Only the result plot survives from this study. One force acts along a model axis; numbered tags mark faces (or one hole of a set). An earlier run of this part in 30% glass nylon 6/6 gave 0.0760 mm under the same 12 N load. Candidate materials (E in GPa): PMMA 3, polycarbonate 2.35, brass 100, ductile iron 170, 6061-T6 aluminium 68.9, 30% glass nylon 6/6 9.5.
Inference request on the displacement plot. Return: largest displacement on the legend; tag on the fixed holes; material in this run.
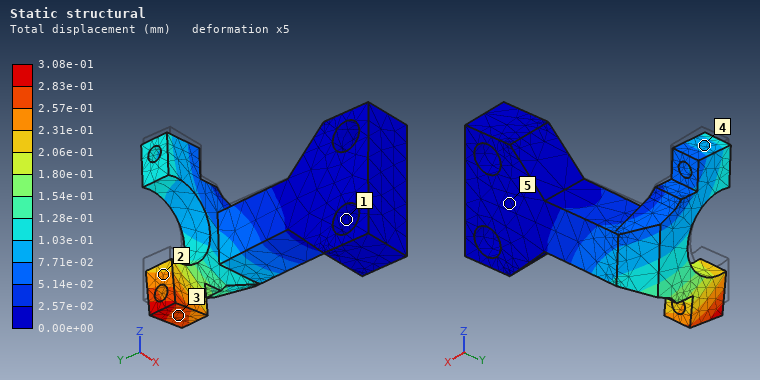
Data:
3.08e-01 mm
1
polycarbonate
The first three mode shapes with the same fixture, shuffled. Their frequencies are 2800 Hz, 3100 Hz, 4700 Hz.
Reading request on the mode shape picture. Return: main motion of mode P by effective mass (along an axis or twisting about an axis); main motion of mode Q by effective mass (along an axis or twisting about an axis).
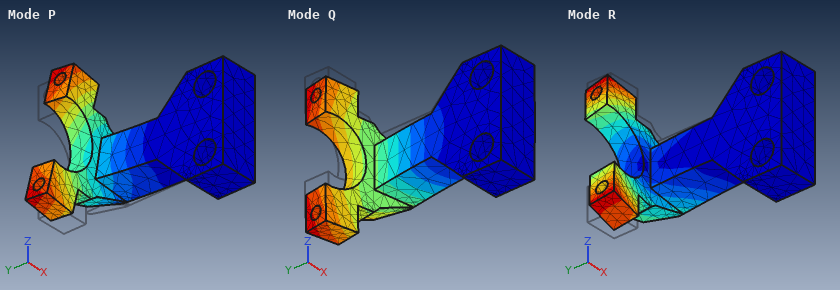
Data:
along Z
along X
